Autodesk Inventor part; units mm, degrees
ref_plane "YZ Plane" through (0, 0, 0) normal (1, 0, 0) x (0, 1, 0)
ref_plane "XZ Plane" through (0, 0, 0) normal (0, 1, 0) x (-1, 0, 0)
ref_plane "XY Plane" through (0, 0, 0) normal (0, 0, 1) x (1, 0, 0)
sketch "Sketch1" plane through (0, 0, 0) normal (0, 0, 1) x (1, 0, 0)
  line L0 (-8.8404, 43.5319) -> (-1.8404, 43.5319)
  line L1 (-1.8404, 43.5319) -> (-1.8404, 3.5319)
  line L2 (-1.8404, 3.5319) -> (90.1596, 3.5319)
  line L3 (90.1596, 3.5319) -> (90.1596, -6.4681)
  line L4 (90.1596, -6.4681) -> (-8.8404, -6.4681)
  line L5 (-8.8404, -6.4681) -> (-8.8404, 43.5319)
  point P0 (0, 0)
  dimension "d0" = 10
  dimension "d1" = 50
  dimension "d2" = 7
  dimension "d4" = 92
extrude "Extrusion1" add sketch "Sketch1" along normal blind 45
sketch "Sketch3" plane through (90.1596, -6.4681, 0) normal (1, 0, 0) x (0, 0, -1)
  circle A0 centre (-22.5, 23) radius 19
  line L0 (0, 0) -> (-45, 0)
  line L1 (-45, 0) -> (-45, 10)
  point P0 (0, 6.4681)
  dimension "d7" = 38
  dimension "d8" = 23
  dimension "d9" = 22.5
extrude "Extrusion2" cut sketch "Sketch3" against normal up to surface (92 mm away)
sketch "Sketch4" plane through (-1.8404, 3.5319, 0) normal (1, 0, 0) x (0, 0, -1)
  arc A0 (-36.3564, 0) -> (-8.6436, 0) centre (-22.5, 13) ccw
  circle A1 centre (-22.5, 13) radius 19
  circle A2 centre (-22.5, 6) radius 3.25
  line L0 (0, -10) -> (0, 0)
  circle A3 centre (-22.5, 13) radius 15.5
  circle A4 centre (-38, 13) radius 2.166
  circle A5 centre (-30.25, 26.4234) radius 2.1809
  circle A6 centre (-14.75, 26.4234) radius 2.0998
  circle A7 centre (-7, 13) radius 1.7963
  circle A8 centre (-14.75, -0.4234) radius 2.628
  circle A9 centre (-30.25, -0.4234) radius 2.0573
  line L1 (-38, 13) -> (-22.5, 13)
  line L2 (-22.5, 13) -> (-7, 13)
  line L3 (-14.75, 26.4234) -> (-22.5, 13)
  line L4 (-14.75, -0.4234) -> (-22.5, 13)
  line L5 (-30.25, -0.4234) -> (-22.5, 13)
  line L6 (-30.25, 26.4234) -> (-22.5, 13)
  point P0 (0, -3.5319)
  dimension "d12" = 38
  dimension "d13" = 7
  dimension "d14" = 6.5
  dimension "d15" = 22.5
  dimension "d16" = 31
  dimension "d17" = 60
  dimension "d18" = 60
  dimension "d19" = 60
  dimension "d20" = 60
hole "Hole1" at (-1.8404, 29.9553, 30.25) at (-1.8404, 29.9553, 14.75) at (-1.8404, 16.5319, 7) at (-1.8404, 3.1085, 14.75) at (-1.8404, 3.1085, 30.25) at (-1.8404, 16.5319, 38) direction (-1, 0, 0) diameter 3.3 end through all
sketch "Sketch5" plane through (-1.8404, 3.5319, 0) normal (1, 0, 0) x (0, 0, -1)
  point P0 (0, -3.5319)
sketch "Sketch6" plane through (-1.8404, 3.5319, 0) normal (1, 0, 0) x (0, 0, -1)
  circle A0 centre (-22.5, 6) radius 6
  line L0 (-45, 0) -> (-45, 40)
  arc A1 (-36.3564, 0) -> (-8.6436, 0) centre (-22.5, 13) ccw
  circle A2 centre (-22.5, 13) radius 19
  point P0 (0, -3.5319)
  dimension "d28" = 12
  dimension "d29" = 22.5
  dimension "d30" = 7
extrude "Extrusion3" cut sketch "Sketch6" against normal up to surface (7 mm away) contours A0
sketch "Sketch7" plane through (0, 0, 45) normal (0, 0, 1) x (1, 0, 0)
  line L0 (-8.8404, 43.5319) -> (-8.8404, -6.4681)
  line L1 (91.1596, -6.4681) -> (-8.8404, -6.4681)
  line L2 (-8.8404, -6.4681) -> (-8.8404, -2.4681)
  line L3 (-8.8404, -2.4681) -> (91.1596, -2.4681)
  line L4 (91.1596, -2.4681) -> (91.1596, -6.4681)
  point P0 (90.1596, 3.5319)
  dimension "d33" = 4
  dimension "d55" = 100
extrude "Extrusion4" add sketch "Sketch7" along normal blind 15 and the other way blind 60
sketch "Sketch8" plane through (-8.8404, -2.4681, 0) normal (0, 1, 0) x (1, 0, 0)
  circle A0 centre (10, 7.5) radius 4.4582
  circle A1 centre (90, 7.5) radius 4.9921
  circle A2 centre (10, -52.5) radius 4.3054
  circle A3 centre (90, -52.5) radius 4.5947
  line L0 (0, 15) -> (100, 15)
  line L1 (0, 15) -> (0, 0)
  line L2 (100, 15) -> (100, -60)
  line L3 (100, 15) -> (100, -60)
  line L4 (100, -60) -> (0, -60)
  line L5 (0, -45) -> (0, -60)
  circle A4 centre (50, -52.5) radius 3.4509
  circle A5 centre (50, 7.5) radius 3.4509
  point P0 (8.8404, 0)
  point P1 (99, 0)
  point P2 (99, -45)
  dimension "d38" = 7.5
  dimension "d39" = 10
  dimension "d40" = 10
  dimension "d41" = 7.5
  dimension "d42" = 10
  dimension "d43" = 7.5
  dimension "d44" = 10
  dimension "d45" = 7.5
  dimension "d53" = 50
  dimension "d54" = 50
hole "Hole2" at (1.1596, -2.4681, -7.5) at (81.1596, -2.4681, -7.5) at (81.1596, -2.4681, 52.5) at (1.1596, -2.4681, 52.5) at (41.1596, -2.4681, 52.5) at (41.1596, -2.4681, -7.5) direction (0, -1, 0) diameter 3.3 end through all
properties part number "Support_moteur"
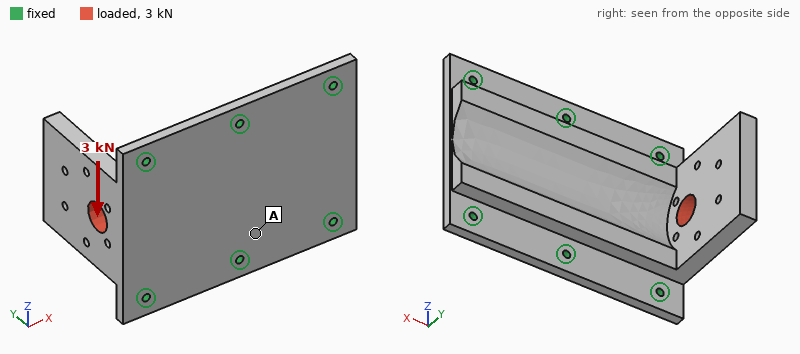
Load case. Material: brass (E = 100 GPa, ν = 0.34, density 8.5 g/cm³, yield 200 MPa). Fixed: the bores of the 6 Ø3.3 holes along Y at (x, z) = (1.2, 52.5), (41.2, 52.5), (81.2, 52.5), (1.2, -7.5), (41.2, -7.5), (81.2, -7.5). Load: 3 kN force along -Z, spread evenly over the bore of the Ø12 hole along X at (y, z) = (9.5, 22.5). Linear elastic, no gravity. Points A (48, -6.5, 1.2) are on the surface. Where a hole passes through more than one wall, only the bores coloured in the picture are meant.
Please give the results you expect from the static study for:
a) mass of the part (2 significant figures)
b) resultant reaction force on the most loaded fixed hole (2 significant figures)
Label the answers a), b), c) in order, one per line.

a) 490 g
b) 1.5 kN
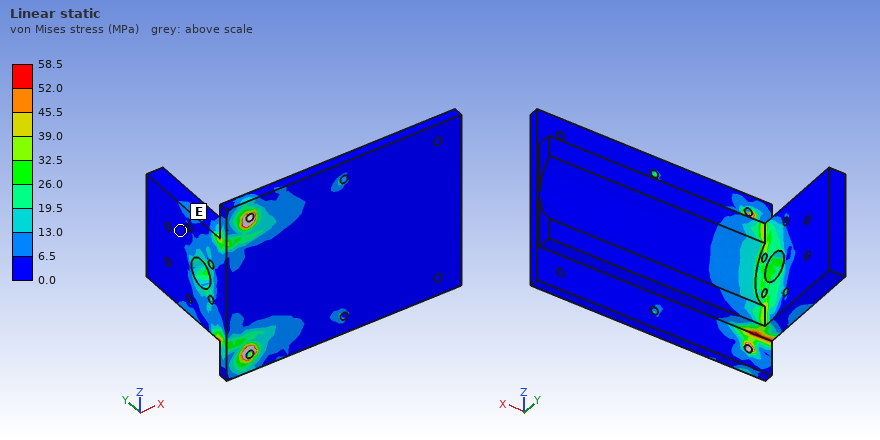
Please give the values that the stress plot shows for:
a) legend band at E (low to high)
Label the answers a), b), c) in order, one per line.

a) 0.0 to 6.5 MPa
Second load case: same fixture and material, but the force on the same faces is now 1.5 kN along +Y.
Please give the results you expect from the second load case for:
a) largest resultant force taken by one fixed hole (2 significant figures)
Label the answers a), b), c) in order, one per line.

a) 960 N
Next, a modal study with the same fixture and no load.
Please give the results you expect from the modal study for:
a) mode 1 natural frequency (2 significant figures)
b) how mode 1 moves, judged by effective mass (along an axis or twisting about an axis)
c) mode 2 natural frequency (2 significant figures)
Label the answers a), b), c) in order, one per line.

a) 1300 Hz
b) along X
c) 3300 Hz
